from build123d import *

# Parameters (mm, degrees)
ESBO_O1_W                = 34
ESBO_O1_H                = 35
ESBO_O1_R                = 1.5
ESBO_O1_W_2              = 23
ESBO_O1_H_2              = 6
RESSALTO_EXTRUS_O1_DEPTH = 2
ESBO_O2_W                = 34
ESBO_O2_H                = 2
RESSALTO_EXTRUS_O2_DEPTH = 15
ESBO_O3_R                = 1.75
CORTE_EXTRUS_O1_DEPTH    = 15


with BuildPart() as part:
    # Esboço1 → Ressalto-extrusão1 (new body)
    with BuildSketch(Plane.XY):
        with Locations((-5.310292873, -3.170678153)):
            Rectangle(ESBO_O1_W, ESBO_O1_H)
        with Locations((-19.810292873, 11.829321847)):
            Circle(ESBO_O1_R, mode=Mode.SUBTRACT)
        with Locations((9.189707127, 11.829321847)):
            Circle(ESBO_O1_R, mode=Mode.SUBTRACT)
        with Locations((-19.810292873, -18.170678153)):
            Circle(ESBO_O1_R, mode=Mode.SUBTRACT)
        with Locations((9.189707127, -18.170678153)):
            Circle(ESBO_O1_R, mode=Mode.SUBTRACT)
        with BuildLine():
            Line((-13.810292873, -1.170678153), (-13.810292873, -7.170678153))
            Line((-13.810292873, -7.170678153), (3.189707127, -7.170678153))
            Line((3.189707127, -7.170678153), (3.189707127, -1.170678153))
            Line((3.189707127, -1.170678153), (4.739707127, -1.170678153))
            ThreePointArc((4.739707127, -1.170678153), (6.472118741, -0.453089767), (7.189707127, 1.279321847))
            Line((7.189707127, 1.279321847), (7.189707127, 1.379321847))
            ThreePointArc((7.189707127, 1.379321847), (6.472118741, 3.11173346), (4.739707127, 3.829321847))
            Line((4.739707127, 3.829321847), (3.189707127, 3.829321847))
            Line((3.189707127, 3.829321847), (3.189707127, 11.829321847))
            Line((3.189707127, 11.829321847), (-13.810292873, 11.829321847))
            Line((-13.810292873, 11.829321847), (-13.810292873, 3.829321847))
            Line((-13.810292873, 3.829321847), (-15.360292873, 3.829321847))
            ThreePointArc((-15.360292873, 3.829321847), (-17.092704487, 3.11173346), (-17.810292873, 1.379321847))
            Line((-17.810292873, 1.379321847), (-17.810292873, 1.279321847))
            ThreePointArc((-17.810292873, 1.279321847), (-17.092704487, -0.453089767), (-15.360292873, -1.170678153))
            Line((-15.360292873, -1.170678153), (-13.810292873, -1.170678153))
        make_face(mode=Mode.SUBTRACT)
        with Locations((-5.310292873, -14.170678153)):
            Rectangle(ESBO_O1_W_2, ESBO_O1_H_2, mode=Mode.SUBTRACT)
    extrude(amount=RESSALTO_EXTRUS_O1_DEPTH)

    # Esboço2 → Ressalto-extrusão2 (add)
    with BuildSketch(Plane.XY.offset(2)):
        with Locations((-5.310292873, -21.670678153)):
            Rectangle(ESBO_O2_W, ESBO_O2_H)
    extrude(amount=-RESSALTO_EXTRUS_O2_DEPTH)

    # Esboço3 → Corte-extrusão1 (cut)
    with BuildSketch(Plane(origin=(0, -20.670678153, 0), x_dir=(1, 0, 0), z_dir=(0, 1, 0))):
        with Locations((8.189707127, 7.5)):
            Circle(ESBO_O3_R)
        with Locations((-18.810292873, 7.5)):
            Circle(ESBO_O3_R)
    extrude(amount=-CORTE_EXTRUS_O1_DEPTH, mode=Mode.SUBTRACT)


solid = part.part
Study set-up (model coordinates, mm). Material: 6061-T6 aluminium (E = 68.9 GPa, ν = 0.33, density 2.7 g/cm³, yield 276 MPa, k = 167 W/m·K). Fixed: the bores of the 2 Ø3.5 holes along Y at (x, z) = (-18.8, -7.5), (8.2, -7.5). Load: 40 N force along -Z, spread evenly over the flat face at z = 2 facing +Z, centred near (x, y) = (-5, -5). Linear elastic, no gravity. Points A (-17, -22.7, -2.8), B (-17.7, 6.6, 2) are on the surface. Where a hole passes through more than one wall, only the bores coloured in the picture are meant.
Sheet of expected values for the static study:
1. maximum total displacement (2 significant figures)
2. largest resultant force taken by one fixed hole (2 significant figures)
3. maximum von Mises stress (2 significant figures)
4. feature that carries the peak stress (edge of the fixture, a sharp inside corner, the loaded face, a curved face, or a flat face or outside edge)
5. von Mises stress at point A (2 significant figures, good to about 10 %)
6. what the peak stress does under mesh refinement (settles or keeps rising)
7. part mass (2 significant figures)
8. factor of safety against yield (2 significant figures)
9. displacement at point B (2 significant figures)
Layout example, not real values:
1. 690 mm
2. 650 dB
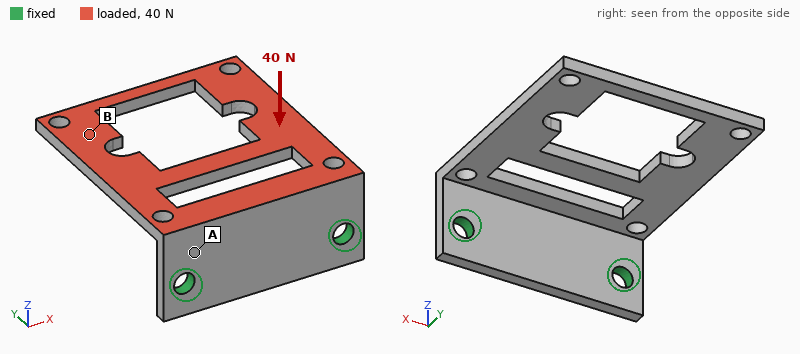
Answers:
1. 0.58 mm
2. 20 N
3. 170 MPa
4. a curved face
5. 32 MPa
6. settles
7. 6.2 g
8. 1.6
9. 0.42 mm
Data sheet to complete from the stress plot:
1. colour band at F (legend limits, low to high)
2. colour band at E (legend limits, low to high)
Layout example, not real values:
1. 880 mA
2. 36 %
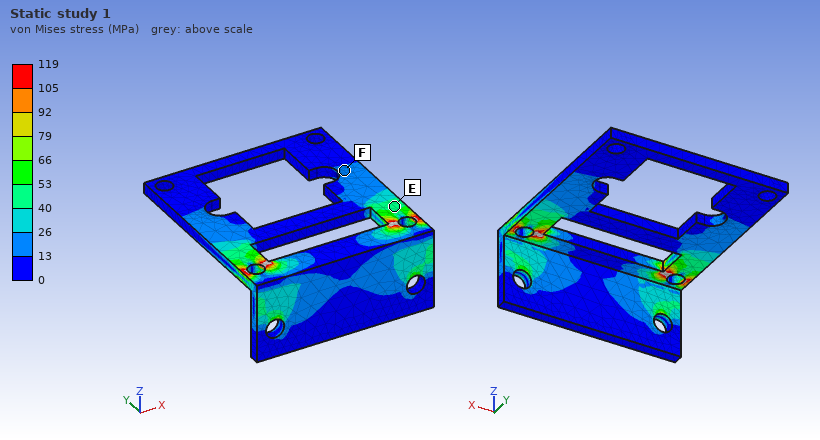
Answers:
1. 13 to 26 MPa
2. 40 to 53 MPa
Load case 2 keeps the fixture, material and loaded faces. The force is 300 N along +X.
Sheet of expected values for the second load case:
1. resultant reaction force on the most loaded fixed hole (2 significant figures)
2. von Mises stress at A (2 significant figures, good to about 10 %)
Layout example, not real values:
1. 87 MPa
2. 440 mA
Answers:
1. 250 N
2. 61 MPa
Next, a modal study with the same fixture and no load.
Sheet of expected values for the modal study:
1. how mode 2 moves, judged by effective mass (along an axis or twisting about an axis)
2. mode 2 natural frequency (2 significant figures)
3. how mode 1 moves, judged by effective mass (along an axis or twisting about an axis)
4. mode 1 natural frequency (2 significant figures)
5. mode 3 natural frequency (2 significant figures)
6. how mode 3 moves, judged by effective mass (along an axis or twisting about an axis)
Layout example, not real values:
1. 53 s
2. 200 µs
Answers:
1. twisting about Y
2. 2100 Hz
3. along Z
4. 810 Hz
5. 3600 Hz
6. along X
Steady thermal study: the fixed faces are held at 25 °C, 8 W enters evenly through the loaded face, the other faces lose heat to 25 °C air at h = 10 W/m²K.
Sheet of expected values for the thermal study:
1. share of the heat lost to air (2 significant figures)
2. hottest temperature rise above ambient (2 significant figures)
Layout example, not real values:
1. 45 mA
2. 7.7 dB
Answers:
1. 4.9 %
2. 41 K
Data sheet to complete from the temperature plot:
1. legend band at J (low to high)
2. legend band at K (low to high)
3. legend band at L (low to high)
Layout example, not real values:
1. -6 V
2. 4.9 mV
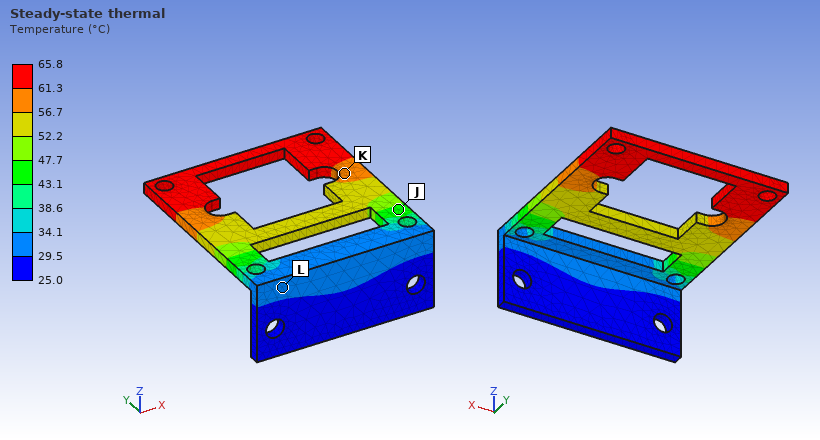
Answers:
1. 43.1 to 47.7 °C
2. 56.7 to 61.3 °C
3. 29.5 to 34.1 °C
